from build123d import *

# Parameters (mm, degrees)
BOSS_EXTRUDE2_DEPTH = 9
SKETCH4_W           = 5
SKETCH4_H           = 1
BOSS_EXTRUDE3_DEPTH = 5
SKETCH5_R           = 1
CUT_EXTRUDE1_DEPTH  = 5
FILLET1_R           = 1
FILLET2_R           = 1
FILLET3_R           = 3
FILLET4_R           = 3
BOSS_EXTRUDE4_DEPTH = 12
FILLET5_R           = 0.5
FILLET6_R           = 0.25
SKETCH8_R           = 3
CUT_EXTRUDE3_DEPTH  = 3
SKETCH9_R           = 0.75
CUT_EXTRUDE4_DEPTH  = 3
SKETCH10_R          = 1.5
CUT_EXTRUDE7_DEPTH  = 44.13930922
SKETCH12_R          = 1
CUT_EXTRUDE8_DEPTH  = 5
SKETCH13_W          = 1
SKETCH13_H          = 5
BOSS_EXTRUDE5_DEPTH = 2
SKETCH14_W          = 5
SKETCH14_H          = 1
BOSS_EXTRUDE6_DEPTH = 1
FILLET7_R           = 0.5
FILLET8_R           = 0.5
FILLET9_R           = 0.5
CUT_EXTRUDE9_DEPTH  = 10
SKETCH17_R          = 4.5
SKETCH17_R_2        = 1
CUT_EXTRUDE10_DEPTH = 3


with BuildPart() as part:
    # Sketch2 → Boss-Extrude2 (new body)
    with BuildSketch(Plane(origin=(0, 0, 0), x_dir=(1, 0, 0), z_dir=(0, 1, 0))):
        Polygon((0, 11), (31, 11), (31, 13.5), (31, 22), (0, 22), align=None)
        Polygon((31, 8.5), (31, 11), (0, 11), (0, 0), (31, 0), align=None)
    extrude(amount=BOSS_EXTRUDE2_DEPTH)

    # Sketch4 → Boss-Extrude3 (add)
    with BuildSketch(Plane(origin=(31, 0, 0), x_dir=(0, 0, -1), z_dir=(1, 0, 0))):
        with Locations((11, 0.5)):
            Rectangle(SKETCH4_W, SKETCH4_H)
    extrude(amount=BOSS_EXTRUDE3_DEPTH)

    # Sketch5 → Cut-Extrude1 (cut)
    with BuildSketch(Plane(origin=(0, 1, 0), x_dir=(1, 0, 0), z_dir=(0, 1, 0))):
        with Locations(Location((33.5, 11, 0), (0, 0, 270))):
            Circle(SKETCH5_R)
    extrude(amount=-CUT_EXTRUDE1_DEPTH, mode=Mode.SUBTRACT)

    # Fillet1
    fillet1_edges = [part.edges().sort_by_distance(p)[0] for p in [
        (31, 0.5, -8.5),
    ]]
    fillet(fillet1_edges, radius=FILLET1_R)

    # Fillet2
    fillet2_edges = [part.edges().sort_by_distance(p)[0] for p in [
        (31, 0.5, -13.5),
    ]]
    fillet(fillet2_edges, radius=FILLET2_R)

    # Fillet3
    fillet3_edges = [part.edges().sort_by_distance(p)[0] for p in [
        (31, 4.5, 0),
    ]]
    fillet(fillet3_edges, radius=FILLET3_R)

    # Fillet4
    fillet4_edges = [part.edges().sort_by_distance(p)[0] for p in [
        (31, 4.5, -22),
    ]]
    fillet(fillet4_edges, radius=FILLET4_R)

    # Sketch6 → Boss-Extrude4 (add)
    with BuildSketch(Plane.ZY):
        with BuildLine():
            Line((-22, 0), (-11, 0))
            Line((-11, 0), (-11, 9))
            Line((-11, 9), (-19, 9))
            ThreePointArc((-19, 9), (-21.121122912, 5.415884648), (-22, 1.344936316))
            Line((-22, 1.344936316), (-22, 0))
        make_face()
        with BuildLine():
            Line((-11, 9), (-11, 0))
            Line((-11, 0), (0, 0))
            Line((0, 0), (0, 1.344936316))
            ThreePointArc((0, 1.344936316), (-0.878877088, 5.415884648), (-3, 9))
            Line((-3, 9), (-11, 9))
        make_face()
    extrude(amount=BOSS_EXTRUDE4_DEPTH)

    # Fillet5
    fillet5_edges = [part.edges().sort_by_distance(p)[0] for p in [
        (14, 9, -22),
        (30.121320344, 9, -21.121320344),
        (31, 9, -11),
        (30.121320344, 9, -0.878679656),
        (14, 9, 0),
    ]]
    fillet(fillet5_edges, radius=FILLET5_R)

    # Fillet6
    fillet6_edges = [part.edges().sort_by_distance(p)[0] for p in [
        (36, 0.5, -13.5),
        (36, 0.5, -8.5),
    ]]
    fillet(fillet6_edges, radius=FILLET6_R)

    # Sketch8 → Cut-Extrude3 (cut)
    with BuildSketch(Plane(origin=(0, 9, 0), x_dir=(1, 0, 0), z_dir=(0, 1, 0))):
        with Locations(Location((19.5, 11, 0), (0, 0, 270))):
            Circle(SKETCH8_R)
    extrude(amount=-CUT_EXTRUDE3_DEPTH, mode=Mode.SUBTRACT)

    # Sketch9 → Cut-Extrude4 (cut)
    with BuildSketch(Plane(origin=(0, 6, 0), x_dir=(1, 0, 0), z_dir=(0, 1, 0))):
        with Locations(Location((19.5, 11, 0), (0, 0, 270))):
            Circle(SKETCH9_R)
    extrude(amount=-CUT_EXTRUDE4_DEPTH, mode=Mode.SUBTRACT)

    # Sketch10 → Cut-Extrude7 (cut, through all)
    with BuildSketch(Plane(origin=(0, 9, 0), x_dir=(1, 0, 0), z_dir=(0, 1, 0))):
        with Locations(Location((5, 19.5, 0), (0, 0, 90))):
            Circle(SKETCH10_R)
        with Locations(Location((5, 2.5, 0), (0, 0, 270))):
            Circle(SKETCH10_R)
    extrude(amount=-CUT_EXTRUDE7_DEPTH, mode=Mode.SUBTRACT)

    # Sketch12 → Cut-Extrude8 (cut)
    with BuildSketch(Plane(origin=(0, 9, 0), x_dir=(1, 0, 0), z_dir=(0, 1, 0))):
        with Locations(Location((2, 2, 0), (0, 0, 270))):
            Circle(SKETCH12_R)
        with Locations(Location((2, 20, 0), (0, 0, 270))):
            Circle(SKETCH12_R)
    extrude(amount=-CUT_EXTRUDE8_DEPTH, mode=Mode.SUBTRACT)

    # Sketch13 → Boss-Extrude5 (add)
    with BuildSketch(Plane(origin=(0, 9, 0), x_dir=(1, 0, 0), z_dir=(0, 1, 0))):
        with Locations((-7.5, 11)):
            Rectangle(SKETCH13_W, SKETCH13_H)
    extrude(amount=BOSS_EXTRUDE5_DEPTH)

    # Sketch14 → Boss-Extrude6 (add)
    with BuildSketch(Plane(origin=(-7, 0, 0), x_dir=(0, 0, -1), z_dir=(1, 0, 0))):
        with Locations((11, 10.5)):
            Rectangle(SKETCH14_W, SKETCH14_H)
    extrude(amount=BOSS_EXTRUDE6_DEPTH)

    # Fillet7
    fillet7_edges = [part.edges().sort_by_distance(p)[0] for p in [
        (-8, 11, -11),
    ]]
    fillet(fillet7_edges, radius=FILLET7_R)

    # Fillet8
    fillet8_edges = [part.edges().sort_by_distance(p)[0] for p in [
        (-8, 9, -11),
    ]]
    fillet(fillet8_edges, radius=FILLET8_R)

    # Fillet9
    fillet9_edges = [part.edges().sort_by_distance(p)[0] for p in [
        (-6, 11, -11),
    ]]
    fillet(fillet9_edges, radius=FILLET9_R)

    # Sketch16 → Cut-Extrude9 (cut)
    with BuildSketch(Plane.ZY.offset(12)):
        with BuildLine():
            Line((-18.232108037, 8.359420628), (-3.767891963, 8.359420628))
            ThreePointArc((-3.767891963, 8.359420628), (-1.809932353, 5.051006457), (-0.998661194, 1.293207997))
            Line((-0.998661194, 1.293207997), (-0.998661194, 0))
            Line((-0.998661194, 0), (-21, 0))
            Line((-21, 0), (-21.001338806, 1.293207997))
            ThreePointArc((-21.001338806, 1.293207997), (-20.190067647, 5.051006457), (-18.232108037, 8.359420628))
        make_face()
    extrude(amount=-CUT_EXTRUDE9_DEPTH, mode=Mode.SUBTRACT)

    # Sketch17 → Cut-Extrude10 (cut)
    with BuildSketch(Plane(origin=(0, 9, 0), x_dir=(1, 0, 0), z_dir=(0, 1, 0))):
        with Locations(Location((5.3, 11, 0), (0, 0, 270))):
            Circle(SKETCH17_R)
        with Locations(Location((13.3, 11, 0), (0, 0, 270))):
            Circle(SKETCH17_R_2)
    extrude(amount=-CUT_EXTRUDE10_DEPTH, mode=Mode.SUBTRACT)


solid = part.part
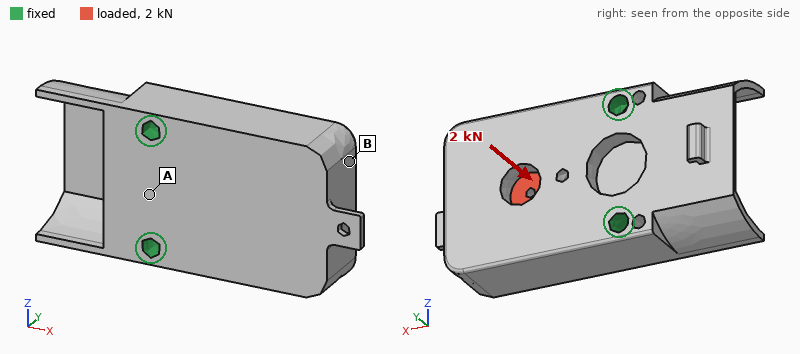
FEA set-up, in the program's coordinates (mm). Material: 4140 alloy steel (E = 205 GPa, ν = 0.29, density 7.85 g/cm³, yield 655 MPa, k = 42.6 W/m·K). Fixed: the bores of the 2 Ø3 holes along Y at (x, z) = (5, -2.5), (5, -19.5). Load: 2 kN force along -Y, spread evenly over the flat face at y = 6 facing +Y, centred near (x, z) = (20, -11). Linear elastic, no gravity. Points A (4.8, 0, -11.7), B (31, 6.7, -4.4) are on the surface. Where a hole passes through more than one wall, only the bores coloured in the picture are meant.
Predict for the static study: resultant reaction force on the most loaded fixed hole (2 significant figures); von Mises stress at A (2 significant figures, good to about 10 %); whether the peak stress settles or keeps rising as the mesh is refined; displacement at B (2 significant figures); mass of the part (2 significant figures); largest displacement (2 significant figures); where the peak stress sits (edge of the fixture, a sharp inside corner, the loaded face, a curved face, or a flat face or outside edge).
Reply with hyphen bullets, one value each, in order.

- 1.0 kN
- 36 MPa
- keeps rising
- 23 µm
- 50 g
- 29 µm
- edge of the fixture
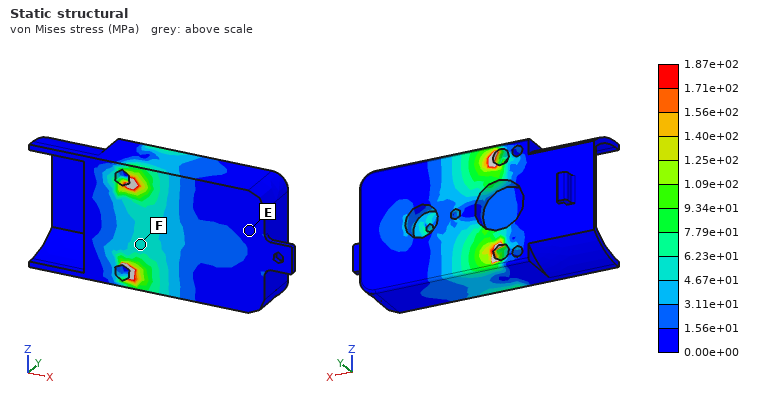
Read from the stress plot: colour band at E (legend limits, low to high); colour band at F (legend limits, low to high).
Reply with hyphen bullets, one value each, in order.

- 0.00e+00 to 1.56e+01 MPa
- 4.67e+01 to 6.23e+01 MPa
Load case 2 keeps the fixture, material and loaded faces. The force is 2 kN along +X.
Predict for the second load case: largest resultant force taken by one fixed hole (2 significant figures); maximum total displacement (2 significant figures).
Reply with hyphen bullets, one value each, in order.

- 1.0 kN
- 5.2 µm
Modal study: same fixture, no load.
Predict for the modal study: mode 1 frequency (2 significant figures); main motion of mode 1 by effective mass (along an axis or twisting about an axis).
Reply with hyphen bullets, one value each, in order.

- 9200 Hz
- along Y
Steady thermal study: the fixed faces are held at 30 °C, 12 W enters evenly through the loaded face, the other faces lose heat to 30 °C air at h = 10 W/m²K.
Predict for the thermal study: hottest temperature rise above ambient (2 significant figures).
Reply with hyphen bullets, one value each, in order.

- 41 K
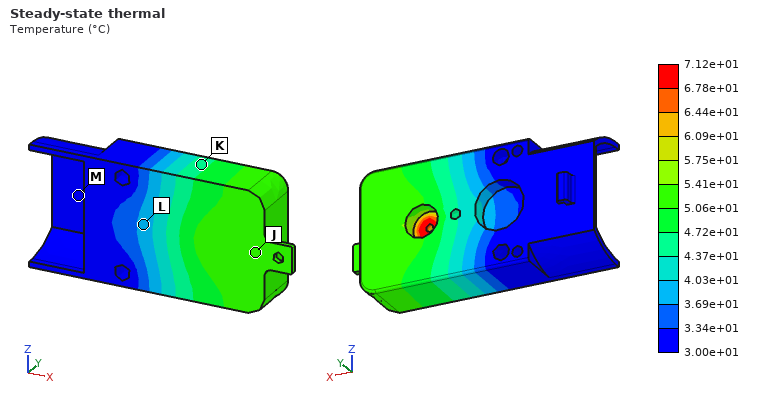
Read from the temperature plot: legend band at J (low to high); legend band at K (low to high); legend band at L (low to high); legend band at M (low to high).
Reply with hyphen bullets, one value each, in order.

- 5.06e+01 to 5.41e+01 °C
- 4.37e+01 to 4.72e+01 °C
- 3.69e+01 to 4.03e+01 °C
- 3.00e+01 to 3.34e+01 °C
